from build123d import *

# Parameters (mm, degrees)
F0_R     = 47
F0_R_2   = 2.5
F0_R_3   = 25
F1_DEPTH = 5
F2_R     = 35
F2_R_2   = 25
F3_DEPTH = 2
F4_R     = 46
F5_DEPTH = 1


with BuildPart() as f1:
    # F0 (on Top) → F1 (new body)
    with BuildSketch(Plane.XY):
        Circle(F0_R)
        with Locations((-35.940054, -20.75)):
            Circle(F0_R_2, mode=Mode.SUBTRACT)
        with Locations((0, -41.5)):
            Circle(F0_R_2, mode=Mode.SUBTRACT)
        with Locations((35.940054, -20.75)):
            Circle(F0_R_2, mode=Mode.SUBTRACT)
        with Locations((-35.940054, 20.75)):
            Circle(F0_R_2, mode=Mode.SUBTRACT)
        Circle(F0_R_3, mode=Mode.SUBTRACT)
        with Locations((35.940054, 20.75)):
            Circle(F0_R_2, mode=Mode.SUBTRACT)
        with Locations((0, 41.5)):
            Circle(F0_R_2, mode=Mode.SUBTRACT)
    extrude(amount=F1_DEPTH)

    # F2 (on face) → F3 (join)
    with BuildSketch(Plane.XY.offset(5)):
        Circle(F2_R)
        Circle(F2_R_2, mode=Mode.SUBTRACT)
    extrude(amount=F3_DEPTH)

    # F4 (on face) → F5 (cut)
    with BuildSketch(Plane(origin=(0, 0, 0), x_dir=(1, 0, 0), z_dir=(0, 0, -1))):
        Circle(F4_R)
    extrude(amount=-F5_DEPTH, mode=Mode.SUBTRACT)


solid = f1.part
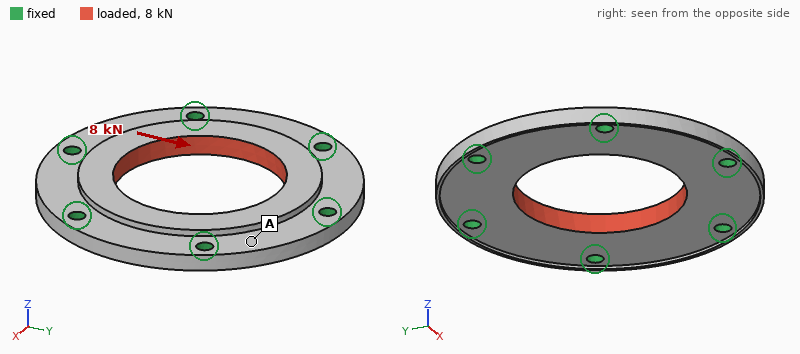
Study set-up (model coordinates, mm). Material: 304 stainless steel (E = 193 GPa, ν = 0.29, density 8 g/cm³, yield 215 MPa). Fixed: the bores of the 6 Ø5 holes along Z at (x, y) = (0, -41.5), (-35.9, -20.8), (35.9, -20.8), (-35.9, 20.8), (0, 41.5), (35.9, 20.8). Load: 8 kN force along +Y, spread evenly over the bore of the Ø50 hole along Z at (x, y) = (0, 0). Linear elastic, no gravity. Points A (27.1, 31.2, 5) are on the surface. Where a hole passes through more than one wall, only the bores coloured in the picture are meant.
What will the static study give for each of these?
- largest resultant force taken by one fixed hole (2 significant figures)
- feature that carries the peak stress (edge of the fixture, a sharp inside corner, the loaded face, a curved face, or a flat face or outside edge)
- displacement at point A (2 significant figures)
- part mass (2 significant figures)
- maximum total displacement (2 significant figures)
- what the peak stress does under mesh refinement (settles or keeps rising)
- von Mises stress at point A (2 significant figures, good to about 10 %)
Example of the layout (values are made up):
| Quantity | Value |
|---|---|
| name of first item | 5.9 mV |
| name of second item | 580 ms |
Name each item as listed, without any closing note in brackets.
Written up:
| Quantity | Value |
|---|---|
| largest resultant force taken by one fixed hole | 1.7 kN |
| feature that carries the peak stress | edge of the fixture |
| displacement at point A | 1.6 µm |
| part mass | 190 g |
| maximum total displacement | 3.6 µm |
| what the peak stress does under mesh refinement | keeps rising |
| von Mises stress at point A | 8.9 MPa |
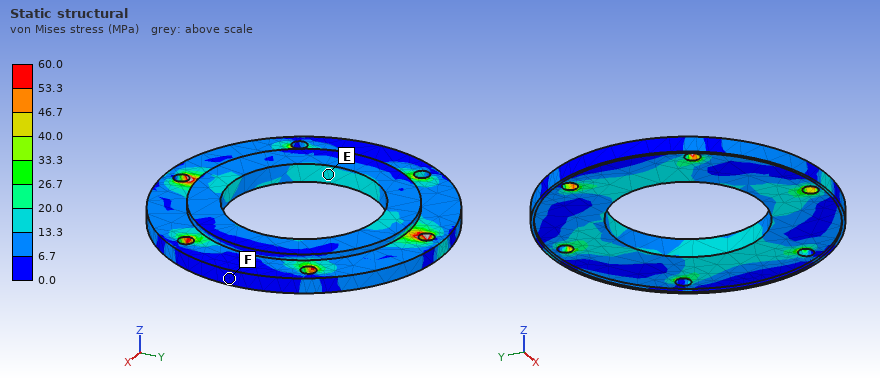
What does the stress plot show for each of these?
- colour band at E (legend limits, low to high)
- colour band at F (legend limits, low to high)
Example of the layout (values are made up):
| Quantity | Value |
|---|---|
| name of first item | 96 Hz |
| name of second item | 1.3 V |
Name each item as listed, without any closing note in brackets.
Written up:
| Quantity | Value |
|---|---|
| colour band at E | 13.3 to 20.0 MPa |
| colour band at F | 0.0 to 6.7 MPa |
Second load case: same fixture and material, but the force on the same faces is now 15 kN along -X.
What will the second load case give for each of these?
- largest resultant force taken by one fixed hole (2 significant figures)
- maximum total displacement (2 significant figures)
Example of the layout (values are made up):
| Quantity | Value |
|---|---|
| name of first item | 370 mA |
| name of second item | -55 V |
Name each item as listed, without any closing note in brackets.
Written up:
| Quantity | Value |
|---|---|
| largest resultant force taken by one fixed hole | 2.8 kN |
| maximum total displacement | 7.5 µm |
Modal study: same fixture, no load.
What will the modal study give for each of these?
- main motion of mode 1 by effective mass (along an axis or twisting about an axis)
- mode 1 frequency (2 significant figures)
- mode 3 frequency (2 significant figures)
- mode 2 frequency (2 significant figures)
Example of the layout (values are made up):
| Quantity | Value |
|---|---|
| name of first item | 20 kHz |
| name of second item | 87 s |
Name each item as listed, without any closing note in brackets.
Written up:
| Quantity | Value |
|---|---|
| main motion of mode 1 by effective mass | along Z |
| mode 1 frequency | 9500 Hz |
| mode 3 frequency | 12 kHz |
| mode 2 frequency | 11 kHz |
